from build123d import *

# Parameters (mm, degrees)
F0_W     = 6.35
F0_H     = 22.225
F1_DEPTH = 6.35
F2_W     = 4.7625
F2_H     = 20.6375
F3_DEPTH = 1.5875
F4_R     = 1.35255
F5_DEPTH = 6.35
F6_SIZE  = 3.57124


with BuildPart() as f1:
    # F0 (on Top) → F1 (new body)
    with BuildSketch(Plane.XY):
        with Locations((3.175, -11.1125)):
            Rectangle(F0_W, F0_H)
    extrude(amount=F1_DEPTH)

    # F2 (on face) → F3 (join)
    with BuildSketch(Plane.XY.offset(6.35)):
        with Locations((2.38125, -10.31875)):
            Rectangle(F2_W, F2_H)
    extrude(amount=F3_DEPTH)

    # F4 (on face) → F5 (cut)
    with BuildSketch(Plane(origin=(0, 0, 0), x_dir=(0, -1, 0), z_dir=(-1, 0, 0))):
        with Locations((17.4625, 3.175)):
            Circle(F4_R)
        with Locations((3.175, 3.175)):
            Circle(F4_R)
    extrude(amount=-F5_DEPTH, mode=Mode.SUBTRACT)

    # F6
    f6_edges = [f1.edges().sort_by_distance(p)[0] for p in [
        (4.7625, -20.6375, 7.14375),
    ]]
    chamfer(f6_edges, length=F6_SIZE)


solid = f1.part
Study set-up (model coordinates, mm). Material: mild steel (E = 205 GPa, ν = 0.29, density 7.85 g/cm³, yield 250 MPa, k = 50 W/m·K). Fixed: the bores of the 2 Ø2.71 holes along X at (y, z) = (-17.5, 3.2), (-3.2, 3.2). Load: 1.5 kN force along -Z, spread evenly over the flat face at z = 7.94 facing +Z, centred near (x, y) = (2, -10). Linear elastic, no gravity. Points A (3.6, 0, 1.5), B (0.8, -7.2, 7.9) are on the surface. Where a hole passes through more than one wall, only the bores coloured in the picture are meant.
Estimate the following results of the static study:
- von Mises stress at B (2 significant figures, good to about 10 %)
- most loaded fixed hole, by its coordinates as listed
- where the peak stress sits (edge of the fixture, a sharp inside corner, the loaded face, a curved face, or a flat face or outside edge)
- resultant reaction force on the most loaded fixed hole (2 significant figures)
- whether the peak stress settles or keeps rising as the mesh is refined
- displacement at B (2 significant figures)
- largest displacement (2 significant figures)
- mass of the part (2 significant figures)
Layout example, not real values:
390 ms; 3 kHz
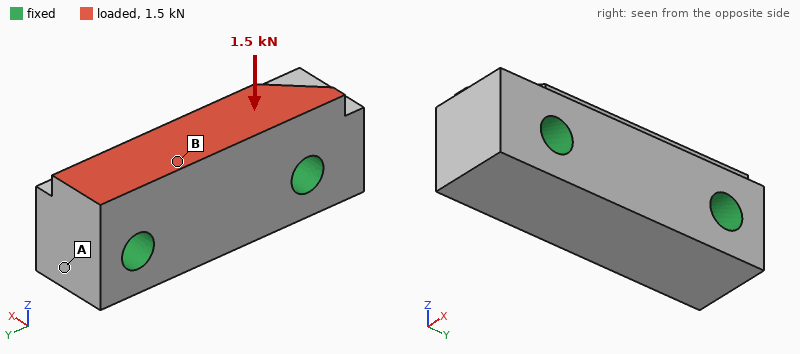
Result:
15 MPa; (-3.2, 3.2); edge of the fixture; 820 N; keeps rising; 0.94 µm; 1.2 µm; 7.6 g
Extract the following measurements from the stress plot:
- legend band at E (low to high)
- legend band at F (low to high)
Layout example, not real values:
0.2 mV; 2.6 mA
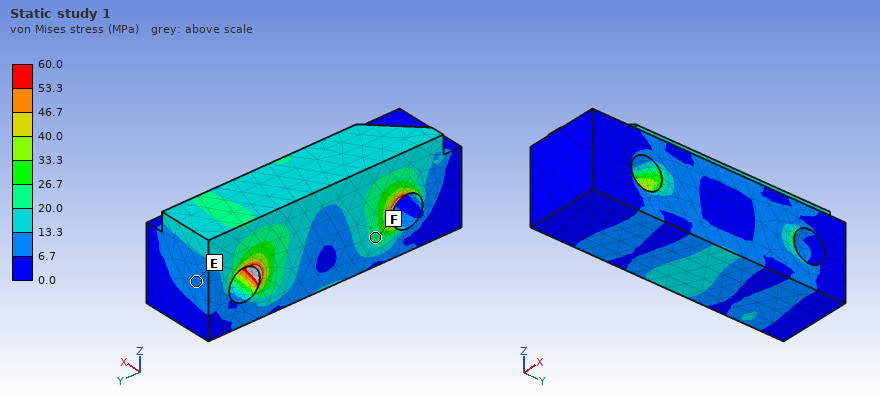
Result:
6.7 to 13.3 MPa; 20.0 to 26.7 MPa
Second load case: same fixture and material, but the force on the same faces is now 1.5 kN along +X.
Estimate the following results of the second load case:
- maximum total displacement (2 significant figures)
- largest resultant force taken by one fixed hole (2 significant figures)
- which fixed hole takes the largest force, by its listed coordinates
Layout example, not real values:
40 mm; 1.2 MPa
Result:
3.6 µm; 800 N; (-3.2, 3.2)
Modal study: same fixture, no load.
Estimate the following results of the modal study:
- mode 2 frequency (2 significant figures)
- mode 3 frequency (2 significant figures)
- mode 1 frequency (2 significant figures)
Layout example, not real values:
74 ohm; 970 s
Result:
90 kHz; 110 kHz; 88 kHz
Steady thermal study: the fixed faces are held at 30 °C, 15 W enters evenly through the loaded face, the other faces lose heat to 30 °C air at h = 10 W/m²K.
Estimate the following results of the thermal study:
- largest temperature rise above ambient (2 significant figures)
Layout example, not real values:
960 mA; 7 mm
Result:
18 K
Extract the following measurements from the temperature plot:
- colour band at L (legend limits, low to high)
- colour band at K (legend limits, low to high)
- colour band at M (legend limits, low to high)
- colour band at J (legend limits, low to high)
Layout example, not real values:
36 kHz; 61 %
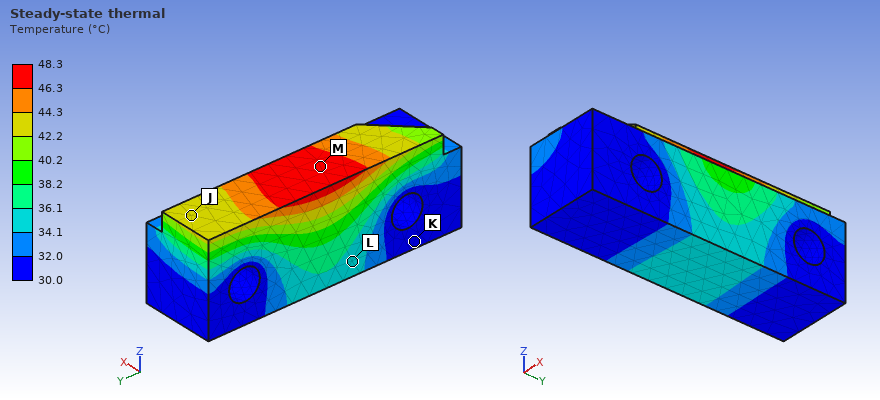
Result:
34.1 to 36.1 °C; 30.0 to 32.0 °C; 46.3 to 48.3 °C; 42.2 to 44.3 °C
